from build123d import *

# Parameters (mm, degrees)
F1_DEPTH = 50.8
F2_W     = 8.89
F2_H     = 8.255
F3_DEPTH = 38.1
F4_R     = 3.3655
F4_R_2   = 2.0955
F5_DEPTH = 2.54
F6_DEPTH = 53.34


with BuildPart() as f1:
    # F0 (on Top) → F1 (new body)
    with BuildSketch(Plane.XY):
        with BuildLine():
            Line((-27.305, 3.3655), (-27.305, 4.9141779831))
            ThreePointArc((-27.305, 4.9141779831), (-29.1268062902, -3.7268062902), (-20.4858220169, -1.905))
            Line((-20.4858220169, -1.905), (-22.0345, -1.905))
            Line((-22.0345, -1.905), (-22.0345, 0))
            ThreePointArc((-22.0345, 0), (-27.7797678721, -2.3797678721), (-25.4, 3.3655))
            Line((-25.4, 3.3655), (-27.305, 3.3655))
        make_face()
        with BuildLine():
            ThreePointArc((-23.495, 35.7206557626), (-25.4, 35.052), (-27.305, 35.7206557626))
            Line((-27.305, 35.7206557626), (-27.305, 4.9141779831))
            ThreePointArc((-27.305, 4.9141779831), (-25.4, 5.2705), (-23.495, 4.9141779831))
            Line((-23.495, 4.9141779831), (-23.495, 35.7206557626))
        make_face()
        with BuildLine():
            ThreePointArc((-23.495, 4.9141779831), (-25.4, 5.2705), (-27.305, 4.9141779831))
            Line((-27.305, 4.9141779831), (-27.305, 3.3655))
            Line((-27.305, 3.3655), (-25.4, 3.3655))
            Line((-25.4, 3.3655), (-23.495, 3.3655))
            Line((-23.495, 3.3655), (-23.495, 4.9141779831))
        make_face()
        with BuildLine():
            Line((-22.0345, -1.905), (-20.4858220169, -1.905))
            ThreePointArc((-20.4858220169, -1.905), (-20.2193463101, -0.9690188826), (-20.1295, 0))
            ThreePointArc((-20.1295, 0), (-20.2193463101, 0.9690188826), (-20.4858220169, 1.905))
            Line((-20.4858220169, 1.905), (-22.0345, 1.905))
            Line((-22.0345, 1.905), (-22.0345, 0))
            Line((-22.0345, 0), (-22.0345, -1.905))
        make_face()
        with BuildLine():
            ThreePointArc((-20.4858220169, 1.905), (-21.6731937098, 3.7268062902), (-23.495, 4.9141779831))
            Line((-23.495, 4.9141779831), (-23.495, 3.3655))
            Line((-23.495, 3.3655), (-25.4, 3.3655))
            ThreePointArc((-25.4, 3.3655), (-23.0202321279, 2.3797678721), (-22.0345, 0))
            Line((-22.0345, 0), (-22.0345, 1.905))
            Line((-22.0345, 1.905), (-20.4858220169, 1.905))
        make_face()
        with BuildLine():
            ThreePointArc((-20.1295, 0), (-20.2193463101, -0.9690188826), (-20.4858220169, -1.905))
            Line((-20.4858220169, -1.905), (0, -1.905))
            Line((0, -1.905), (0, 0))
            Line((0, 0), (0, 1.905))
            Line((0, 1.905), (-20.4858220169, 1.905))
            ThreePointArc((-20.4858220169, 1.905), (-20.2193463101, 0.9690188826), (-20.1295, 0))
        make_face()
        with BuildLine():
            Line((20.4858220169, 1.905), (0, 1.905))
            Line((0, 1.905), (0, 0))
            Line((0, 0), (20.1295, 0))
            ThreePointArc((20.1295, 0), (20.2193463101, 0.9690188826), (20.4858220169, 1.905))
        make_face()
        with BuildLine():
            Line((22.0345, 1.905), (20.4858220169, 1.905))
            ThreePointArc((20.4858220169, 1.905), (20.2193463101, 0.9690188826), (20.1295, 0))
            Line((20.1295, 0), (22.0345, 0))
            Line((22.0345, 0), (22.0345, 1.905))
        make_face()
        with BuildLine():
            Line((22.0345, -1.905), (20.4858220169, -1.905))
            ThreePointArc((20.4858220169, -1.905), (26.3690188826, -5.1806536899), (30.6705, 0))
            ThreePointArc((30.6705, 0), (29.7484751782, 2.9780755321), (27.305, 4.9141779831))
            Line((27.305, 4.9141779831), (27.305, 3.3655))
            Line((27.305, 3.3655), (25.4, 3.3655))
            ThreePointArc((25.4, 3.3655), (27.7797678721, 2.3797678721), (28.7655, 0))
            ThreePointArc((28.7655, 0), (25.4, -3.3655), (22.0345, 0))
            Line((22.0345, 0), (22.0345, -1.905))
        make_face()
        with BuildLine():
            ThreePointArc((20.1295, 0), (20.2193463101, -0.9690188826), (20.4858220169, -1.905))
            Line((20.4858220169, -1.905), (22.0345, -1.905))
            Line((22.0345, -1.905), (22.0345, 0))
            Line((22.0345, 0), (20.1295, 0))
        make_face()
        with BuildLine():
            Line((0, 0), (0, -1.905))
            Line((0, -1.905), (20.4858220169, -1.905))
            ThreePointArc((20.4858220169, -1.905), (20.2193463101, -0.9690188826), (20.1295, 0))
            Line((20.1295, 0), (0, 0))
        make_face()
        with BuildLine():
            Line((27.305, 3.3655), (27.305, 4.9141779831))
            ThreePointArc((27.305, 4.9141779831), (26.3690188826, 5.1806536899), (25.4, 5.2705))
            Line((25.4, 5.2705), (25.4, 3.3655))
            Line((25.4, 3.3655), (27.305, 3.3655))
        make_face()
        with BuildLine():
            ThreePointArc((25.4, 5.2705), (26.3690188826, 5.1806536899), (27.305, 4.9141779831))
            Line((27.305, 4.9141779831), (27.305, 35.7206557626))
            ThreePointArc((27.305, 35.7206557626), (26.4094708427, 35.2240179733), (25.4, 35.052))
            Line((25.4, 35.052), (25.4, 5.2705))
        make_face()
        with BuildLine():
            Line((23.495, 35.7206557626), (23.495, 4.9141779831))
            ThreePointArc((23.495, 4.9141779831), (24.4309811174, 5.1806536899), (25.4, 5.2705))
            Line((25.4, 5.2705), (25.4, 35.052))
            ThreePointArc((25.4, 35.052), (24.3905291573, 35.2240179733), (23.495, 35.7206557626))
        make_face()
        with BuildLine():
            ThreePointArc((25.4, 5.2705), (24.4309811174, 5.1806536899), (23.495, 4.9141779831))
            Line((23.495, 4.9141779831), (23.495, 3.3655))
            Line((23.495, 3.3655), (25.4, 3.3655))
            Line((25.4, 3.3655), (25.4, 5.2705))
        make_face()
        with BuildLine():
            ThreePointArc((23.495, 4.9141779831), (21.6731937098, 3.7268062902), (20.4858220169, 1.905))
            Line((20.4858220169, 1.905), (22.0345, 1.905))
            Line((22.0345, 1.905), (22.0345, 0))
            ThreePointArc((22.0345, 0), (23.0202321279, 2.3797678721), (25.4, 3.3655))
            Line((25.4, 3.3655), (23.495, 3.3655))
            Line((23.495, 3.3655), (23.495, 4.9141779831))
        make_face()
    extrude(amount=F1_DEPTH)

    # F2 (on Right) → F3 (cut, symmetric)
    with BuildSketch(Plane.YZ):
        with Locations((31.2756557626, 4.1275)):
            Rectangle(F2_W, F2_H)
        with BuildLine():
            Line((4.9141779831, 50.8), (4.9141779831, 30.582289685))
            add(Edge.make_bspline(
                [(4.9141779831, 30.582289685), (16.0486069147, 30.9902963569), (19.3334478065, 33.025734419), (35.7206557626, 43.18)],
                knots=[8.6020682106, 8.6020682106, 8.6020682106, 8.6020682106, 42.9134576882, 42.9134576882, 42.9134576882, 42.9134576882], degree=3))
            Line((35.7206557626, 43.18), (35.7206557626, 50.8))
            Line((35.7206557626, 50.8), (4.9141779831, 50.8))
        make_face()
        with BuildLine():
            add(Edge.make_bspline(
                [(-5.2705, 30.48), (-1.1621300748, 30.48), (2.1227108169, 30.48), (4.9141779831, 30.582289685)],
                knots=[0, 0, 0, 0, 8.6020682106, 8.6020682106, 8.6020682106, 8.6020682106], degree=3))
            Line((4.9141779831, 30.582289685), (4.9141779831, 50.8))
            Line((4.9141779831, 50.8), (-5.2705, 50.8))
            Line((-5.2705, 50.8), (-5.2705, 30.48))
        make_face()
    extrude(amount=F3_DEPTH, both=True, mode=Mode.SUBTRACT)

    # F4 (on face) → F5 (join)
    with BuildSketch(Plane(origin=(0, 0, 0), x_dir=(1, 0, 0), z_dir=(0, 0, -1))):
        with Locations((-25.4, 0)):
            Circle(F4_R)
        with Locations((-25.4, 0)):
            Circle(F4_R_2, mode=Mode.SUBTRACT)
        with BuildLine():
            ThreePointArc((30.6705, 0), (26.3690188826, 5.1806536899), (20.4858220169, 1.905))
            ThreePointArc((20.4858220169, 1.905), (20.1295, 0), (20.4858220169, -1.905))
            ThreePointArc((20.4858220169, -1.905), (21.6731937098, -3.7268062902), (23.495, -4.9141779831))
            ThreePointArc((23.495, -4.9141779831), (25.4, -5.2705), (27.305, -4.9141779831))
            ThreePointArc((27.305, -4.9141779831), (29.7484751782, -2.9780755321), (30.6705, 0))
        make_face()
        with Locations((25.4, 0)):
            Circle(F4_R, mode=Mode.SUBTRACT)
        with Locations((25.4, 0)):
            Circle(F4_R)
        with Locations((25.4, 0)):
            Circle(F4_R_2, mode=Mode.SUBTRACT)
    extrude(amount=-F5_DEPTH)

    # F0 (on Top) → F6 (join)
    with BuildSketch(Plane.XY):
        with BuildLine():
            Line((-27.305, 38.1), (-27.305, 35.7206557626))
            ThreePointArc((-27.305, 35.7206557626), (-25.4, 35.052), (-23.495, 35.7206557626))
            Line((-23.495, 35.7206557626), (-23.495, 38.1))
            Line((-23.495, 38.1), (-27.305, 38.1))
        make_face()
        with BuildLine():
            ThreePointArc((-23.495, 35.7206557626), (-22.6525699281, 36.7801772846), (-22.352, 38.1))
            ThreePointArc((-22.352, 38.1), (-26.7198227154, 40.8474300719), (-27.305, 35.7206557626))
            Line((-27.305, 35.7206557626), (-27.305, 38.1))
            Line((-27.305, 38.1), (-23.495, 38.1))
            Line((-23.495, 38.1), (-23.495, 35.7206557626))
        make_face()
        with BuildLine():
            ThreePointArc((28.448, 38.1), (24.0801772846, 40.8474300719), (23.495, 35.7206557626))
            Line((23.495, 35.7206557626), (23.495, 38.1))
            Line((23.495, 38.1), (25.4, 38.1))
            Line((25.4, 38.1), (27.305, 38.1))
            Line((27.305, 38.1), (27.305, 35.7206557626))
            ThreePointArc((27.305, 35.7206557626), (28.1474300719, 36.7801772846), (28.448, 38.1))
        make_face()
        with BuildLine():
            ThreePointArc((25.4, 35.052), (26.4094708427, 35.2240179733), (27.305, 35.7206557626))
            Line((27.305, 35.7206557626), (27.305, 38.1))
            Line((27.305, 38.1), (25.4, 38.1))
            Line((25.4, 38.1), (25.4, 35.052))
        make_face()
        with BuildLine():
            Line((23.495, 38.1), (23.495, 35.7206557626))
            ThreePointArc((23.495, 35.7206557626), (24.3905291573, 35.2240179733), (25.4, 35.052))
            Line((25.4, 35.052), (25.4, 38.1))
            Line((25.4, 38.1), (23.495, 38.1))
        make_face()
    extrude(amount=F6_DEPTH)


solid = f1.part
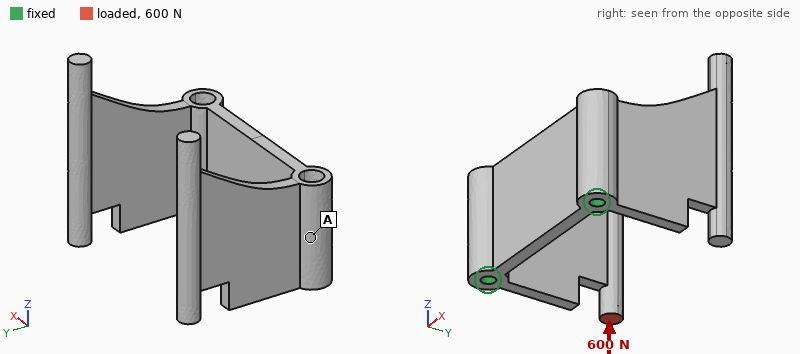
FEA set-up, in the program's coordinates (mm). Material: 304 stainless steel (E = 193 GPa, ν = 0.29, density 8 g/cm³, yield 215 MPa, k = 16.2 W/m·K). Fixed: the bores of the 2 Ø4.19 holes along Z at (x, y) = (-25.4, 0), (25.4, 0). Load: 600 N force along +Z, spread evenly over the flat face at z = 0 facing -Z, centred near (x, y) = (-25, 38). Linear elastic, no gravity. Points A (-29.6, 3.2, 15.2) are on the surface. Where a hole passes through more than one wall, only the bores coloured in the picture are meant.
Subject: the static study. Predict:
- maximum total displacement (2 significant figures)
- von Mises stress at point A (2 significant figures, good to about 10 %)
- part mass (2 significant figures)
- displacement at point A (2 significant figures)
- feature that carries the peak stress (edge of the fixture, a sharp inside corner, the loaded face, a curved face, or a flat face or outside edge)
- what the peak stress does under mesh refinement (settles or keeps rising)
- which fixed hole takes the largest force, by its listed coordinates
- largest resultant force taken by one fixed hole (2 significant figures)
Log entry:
0.25 mm
44 MPa
150 g
0.052 mm
edge of the fixture
keeps rising
(-25.4, 0)
610 N
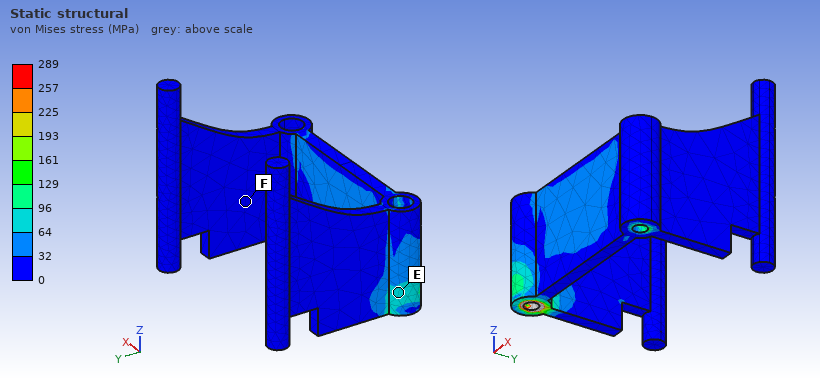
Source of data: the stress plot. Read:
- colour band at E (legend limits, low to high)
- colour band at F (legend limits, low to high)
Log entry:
64 to 96 MPa
0 to 32 MPa
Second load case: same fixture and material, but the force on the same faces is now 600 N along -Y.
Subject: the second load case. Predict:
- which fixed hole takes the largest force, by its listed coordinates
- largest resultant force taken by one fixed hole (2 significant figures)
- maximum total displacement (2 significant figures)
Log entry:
(-25.4, 0)
600 N
40 µm
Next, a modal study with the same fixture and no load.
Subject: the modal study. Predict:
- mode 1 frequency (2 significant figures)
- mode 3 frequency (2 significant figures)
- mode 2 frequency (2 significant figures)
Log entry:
1200 Hz
1400 Hz
1200 Hz
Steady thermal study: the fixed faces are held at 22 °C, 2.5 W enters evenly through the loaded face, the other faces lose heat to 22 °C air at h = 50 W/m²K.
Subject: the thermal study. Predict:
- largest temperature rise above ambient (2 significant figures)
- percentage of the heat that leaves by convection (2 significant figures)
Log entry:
81 K
89 %
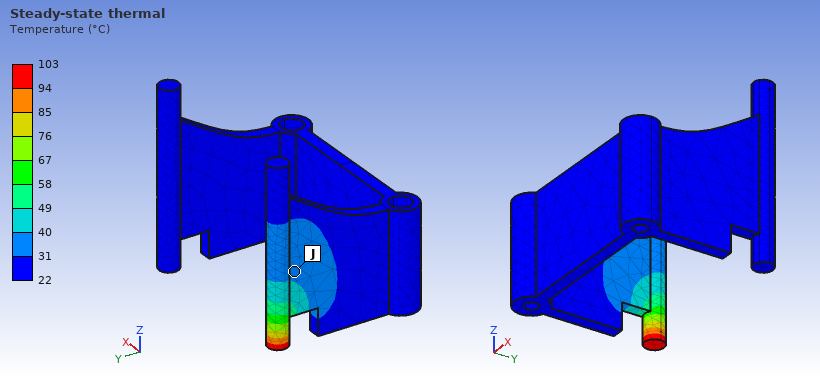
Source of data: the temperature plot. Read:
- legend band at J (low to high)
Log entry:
31 to 40 °C
